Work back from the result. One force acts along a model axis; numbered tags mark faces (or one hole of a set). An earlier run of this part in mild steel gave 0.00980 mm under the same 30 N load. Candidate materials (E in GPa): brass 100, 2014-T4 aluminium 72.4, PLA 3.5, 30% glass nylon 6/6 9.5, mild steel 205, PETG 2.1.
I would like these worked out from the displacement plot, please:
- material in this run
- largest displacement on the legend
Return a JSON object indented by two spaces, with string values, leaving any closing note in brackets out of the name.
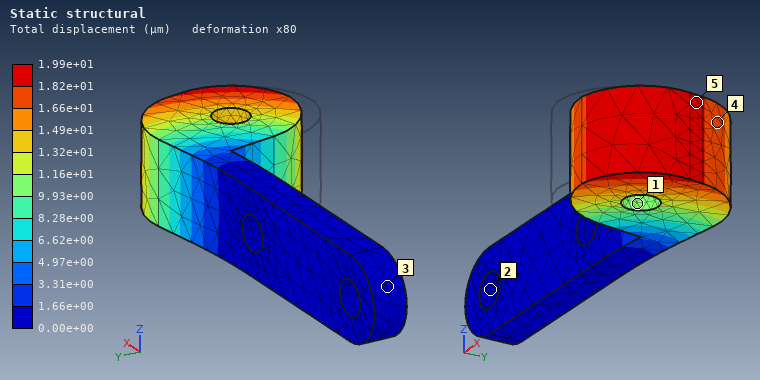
{
  "material in this run": "brass",
  "largest displacement on the legend": "1.99e+01 µm"
}
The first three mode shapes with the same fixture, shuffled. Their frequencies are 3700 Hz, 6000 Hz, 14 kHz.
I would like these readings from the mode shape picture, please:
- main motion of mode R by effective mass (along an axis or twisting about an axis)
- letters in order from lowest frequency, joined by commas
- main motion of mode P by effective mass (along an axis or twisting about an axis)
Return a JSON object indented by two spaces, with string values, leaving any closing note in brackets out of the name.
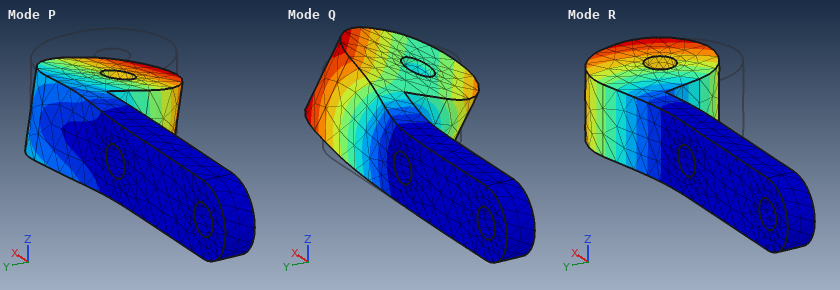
{
  "main motion of mode R by effective mass": "along Y",
  "letters in order from lowest frequency, joined by commas": "R, P, Q",
  "main motion of mode P by effective mass": "along Z"
}
